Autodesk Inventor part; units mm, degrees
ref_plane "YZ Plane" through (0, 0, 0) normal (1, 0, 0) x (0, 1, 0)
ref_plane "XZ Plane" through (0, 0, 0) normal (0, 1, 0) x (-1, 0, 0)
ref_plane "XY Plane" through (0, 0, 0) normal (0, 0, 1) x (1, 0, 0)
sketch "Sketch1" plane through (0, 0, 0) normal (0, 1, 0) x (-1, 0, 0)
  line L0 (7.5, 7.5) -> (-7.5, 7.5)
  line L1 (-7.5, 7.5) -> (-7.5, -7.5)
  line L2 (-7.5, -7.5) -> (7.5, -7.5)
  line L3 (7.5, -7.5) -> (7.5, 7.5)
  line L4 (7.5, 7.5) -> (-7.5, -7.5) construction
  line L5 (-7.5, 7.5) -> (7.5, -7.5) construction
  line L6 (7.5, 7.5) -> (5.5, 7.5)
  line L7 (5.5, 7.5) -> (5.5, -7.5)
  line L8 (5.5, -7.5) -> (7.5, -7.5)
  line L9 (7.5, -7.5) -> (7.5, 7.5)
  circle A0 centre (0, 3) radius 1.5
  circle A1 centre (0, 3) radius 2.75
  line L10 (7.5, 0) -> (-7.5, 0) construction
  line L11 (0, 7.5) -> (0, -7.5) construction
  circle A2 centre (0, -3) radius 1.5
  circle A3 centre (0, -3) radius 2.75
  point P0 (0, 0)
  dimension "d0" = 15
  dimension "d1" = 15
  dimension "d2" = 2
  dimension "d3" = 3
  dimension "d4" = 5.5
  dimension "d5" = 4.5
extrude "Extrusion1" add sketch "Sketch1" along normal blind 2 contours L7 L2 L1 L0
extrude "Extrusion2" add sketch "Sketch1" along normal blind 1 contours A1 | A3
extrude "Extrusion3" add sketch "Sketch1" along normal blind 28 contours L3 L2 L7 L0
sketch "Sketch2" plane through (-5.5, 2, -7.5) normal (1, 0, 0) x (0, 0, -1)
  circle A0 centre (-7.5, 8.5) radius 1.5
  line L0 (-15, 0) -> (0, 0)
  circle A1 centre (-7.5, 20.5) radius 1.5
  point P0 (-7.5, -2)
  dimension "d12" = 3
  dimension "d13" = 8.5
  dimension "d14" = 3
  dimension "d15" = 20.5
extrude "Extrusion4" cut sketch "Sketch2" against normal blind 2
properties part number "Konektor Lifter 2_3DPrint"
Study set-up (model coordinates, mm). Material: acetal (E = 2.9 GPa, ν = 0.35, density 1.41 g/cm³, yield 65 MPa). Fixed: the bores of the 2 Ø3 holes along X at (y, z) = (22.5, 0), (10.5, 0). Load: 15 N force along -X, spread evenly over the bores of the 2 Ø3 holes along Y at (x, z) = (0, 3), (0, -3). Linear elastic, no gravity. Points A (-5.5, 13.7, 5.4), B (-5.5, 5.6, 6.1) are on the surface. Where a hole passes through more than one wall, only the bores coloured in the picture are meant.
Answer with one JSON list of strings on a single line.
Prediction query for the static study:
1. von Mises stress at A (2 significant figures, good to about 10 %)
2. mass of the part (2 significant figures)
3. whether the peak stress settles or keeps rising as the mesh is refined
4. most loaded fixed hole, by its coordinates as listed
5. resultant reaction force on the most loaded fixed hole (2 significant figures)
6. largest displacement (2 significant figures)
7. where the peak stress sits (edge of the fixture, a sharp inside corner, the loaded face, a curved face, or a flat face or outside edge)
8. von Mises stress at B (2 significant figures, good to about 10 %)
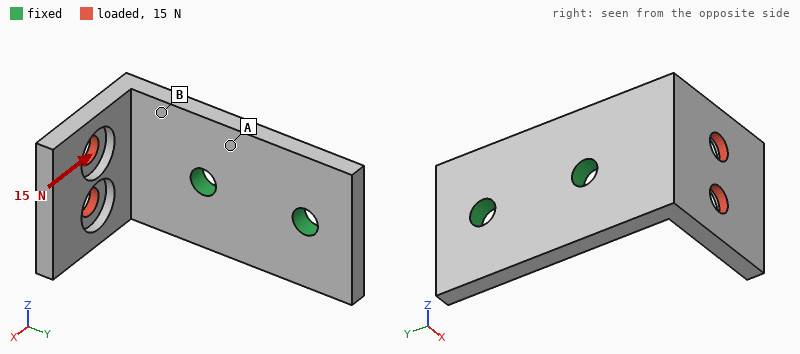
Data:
["2.1 MPa", "1.6 g", "keeps rising", "(10.5, 0)", "18 N", "0.38 mm", "edge of the fixture", "6.5 MPa"]
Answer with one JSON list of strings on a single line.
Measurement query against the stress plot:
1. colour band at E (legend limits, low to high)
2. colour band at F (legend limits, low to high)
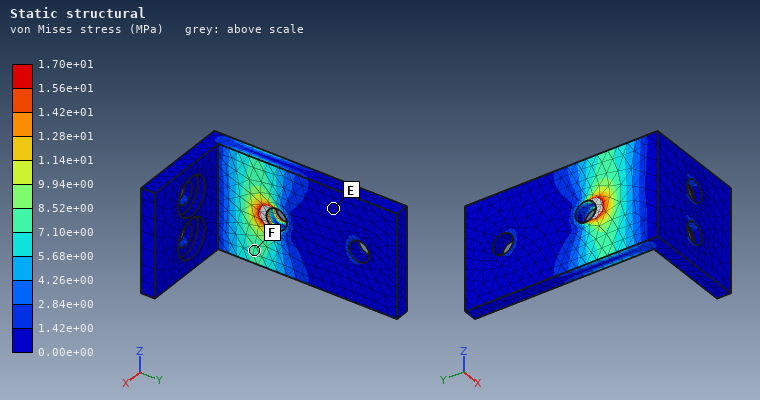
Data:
["0.00e+00 to 1.42e+00 MPa", "7.10e+00 to 8.52e+00 MPa"]
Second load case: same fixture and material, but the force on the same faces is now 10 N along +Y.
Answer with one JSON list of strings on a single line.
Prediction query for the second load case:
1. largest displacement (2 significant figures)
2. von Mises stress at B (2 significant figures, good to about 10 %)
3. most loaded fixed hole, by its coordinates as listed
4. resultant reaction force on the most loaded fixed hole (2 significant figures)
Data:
["0.37 mm", "6.0 MPa", "(10.5, 0)", "8.5 N"]
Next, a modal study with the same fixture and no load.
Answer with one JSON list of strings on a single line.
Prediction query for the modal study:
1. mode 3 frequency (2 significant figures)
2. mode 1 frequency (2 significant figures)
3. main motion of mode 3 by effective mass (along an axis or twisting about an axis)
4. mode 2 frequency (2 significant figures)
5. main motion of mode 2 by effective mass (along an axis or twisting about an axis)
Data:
["3100 Hz", "1200 Hz", "along X", "1700 Hz", "along Z"]
